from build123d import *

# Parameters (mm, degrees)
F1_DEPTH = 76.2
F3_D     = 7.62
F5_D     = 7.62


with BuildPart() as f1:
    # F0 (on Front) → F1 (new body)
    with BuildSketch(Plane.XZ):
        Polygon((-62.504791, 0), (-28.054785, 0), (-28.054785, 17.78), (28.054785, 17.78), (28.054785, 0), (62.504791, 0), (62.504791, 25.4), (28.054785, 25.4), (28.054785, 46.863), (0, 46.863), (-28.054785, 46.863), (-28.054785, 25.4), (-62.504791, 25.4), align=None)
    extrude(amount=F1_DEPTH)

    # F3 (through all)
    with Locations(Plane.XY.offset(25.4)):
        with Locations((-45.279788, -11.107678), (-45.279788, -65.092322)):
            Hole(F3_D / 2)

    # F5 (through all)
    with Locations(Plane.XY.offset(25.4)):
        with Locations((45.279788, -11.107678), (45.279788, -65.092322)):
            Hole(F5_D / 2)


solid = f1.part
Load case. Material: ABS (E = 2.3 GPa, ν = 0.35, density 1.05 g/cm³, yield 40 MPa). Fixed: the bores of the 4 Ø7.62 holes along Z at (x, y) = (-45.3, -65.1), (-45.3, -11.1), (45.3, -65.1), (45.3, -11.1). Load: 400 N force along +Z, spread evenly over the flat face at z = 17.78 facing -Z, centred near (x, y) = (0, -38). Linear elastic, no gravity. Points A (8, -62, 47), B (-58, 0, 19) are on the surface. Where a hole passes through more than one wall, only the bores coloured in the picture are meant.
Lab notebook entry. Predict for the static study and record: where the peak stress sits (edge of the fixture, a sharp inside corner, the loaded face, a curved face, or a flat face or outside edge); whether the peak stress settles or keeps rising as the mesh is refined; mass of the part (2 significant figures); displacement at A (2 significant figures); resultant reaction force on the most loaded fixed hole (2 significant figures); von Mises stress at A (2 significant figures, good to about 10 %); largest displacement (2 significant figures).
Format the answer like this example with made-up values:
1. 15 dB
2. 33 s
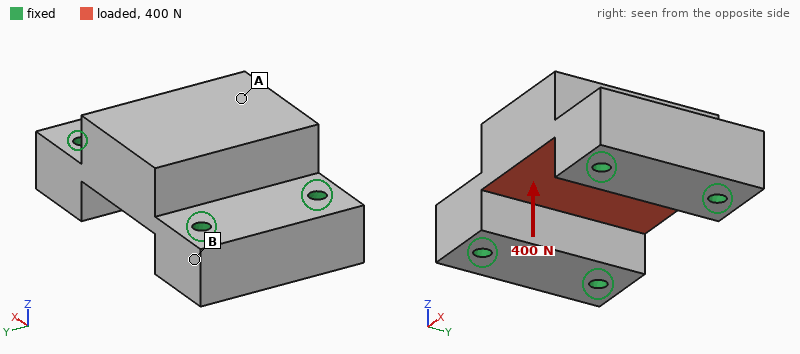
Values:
1. edge of the fixture
2. keeps rising
3. 270 g
4. 9.1 µm
5. 120 N
6. 0.16 MPa
7. 11 µm
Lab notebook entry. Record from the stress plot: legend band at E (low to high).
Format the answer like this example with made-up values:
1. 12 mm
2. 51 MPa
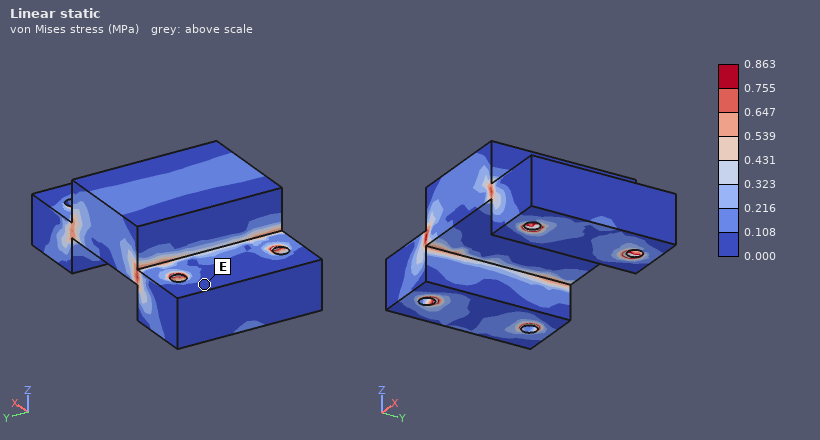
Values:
1. 0.000 to 0.108 MPa
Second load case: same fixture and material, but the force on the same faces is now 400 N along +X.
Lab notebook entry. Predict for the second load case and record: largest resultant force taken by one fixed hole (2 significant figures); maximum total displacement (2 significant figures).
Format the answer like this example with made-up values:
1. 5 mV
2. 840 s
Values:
1. 100 N
2. 5.7 µm
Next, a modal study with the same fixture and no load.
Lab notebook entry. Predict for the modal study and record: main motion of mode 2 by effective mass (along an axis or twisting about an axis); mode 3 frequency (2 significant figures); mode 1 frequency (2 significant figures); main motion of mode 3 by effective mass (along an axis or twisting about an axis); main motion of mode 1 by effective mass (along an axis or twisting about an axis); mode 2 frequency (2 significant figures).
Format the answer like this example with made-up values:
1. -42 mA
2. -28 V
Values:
1. along Z
2. 3800 Hz
3. 2400 Hz
4. along Y
5. along Y
6. 2800 Hz
